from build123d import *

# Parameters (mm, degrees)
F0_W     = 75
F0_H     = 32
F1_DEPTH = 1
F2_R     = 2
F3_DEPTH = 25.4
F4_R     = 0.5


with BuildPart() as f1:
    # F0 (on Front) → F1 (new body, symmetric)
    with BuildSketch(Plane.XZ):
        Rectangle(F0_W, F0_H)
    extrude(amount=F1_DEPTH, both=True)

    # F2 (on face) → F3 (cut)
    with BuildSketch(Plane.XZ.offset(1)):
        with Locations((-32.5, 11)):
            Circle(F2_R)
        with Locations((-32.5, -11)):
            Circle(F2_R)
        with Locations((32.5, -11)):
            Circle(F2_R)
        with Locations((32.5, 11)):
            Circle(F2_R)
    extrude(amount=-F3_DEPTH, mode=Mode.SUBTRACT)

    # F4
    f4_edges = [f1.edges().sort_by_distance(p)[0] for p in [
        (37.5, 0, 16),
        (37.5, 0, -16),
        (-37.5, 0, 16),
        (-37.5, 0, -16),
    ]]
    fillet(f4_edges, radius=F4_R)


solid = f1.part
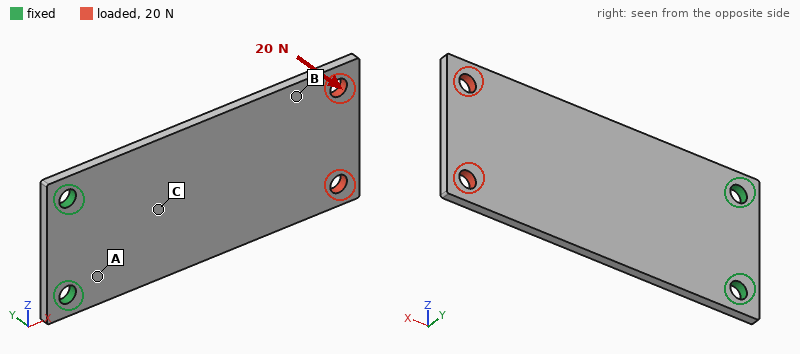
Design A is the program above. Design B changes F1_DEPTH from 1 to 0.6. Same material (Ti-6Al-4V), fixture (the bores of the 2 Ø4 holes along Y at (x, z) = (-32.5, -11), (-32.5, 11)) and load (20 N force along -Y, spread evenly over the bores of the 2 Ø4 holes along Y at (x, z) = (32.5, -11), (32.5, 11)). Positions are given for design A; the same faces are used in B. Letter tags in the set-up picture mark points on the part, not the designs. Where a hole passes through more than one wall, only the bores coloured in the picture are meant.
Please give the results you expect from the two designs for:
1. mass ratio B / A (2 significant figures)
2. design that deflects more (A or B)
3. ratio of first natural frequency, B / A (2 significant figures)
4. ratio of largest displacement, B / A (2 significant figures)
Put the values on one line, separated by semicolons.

0.60; B; 0.61; 4.6
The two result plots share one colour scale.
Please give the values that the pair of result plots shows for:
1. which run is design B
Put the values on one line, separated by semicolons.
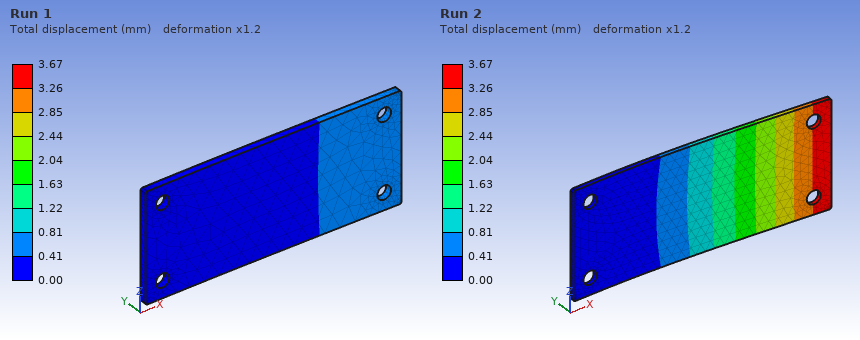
Run 2
